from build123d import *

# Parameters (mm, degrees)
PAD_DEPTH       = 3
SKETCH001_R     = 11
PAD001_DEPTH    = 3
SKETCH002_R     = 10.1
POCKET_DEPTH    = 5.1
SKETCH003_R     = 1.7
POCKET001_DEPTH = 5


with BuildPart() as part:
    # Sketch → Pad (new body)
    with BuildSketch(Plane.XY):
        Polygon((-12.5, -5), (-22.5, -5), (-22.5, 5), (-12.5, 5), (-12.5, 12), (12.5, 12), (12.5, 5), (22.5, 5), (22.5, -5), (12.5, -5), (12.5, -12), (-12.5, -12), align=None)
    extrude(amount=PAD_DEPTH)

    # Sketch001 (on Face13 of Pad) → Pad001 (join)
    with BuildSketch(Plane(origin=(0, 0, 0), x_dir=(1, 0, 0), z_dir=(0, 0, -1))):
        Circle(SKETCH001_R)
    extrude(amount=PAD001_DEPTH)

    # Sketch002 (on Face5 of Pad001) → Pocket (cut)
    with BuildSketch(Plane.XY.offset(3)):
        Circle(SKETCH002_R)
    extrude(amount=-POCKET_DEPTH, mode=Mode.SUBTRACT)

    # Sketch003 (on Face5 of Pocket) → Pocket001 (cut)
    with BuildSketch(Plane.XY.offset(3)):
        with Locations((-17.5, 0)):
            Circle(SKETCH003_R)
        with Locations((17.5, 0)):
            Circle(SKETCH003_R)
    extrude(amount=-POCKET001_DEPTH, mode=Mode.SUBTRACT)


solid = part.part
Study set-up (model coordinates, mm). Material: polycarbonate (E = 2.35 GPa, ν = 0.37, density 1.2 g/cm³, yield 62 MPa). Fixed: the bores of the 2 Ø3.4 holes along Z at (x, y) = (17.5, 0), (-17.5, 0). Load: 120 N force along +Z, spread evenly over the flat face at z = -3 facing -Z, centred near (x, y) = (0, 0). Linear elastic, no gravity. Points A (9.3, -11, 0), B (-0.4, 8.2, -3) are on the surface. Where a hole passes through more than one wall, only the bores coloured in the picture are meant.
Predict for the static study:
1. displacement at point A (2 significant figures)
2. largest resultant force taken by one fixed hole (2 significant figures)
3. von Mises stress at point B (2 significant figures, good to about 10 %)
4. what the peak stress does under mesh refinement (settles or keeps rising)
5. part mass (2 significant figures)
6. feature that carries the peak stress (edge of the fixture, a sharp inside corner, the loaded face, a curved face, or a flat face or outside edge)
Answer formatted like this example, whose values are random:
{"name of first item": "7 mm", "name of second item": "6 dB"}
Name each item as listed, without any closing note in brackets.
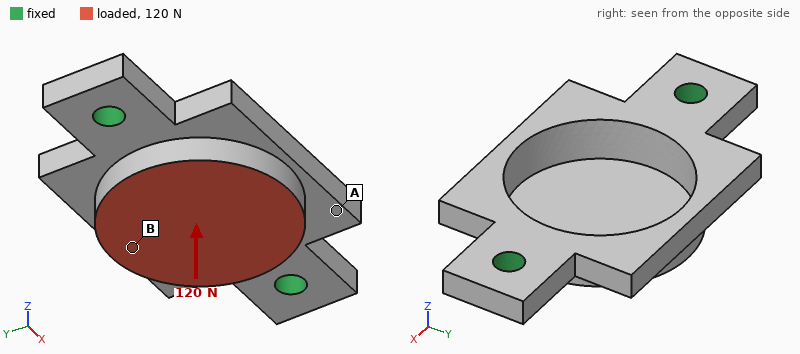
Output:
{"displacement at point A": "0.14 mm", "largest resultant force taken by one fixed hole": "86 N", "von Mises stress at point B": "15 MPa", "what the peak stress does under mesh refinement": "keeps rising", "part mass": "2.2 g", "feature that carries the peak stress": "edge of the fixture"}
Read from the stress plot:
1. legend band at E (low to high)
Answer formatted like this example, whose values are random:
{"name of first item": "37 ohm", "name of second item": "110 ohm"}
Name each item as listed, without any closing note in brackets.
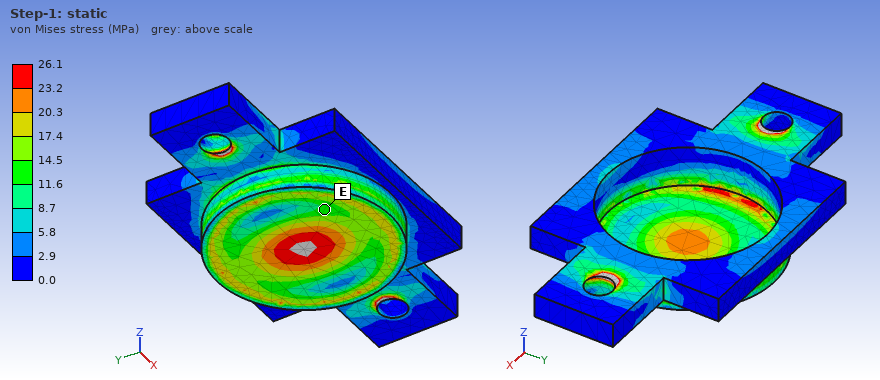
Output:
{"legend band at E": "11.6 to 14.5 MPa"}
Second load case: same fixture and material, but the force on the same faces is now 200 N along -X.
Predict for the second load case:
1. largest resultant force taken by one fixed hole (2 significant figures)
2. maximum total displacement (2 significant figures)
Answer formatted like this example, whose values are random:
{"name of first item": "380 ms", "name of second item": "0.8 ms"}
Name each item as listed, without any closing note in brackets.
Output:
{"largest resultant force taken by one fixed hole": "110 N", "maximum total displacement": "0.10 mm"}
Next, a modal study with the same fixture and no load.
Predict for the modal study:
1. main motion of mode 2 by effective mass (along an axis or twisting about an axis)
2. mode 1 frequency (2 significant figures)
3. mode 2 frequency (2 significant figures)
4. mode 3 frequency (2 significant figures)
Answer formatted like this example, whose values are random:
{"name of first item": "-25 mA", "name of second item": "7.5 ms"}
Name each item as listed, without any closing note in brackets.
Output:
{"main motion of mode 2 by effective mass": "along Z", "mode 1 frequency": "2300 Hz", "mode 2 frequency": "3600 Hz", "mode 3 frequency": "5300 Hz"}
